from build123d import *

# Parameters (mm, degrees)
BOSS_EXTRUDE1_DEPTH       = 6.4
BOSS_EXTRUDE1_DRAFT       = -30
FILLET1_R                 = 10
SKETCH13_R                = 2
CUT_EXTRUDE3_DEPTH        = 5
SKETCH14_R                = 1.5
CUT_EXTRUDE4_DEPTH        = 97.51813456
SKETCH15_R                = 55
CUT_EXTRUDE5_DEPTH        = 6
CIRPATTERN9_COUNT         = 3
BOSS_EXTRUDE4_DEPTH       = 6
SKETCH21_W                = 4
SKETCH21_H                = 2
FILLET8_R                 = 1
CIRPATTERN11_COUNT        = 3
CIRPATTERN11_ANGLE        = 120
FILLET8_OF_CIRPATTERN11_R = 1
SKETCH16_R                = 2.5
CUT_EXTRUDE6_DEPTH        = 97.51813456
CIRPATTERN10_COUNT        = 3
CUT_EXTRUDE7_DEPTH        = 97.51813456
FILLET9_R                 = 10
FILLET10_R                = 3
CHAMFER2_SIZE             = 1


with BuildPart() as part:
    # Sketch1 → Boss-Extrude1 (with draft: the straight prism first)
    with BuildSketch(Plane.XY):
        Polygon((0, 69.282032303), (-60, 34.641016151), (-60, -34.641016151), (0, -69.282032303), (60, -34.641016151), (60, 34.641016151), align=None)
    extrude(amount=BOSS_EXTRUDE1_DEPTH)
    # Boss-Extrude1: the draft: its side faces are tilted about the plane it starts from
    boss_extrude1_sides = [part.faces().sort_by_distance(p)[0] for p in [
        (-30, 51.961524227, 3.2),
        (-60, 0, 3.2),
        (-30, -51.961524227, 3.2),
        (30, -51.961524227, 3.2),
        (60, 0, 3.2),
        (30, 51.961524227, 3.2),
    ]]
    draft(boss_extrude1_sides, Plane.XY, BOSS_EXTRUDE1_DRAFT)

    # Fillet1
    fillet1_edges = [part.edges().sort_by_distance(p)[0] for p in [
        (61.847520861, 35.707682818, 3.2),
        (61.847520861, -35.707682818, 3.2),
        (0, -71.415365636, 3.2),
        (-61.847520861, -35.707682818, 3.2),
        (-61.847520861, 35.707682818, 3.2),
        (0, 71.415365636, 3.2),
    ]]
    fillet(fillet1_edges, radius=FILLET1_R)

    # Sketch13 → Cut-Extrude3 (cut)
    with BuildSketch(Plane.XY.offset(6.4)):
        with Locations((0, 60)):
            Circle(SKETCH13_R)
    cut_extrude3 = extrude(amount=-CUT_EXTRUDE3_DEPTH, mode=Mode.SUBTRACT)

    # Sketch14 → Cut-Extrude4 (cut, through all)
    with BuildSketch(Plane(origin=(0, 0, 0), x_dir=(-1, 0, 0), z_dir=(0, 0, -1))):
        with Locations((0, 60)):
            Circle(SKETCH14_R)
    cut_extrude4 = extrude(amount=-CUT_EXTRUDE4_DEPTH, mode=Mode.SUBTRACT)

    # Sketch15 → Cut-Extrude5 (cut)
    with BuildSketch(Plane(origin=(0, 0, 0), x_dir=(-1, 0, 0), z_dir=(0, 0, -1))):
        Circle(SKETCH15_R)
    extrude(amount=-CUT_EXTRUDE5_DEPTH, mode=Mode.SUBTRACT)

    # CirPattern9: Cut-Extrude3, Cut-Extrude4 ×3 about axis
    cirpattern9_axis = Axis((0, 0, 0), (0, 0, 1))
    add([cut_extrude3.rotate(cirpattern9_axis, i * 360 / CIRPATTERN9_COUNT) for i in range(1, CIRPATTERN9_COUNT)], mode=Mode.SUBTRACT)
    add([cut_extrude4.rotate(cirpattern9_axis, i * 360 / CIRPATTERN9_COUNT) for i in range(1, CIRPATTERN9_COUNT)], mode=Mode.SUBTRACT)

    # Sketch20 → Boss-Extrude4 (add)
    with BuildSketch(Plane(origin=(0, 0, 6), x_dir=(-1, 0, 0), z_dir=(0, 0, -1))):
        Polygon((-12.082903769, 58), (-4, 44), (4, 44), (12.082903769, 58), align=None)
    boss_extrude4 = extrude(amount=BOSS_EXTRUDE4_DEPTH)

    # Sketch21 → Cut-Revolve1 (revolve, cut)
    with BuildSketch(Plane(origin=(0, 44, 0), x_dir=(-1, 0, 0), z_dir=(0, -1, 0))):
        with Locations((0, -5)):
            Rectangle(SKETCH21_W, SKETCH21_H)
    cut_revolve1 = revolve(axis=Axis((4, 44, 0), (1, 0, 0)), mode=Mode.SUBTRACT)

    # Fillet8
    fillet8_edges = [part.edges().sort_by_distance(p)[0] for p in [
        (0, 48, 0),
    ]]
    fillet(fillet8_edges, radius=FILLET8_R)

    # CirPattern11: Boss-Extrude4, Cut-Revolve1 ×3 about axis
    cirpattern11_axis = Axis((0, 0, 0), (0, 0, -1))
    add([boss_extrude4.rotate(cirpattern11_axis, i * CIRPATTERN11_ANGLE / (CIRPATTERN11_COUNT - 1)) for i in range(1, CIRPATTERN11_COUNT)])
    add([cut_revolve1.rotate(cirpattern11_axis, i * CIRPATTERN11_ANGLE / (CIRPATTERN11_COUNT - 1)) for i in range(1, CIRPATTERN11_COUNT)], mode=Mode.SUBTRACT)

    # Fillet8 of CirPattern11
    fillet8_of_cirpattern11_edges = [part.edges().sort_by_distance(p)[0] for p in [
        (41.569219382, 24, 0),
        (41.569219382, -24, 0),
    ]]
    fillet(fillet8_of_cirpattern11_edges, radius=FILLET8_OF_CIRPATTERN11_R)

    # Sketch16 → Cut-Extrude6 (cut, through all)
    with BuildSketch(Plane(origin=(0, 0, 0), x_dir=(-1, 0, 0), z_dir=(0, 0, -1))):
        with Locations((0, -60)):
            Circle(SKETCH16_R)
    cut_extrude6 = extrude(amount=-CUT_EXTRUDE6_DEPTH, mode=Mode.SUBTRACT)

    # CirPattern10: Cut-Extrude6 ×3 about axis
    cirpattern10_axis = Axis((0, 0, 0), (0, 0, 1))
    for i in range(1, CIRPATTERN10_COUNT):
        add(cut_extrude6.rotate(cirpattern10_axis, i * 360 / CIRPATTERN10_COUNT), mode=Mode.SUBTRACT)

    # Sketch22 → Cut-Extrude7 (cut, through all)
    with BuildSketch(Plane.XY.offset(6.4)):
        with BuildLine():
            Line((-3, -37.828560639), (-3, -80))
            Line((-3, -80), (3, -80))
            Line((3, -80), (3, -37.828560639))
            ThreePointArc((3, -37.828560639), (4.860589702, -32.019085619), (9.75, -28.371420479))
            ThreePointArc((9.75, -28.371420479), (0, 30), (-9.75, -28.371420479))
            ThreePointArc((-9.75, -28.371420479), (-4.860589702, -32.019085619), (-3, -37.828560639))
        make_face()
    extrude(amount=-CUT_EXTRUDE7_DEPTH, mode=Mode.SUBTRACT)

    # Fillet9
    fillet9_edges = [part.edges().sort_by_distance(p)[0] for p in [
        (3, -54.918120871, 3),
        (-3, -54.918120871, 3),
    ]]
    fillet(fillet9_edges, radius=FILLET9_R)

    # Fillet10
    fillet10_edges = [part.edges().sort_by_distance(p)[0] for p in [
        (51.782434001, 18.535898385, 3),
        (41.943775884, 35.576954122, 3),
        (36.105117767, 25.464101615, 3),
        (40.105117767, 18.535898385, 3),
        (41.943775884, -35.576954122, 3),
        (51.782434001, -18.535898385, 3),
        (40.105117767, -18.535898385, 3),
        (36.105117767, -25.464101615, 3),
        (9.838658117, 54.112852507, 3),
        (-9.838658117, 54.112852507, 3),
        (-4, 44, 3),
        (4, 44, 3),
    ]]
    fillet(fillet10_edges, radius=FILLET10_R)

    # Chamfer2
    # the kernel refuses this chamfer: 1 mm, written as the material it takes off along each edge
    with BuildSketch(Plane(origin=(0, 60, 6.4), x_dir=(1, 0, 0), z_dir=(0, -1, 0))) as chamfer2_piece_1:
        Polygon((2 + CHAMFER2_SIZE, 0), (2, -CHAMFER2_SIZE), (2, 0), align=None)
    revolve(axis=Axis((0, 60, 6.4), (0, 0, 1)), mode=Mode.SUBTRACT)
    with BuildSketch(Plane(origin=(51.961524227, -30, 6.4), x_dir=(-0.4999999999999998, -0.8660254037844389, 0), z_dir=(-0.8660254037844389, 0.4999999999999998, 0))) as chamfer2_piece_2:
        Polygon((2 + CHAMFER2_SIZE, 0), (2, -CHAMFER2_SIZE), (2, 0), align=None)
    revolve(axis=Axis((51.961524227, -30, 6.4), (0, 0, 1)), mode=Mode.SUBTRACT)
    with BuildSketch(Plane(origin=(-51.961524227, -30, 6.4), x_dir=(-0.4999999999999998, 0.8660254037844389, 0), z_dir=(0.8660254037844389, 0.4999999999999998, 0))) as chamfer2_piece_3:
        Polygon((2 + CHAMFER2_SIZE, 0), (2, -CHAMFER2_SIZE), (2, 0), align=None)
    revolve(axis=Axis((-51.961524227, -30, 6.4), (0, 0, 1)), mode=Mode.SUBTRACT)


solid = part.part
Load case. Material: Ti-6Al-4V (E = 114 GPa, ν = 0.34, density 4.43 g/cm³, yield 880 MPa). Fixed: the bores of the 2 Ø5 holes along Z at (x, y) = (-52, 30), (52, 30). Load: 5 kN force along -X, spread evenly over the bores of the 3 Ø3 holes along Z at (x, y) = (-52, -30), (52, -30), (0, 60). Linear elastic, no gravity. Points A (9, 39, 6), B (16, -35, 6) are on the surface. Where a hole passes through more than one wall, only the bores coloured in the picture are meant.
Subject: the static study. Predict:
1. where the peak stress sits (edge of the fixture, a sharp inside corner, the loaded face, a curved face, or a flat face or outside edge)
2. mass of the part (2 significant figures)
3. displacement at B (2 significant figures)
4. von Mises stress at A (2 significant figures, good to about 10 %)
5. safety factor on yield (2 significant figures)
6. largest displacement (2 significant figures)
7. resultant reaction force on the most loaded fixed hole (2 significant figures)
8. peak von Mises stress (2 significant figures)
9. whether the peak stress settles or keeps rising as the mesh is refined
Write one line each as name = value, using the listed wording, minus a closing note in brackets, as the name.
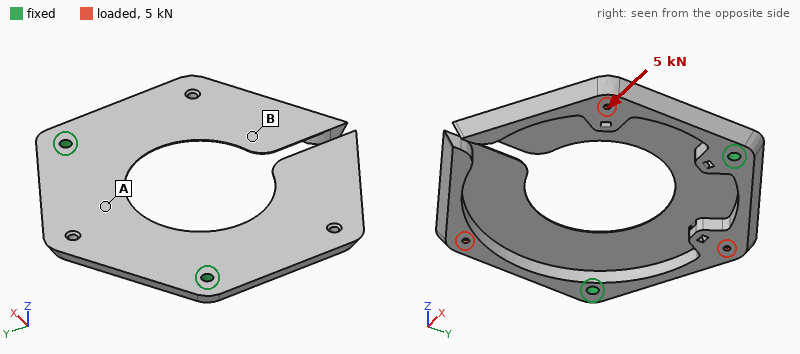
where the peak stress sits = a curved face
mass of the part = 120 g
displacement at B = 0.75 mm
von Mises stress at A = 160 MPa
safety factor on yield = 1.2
largest displacement = 1.2 mm
resultant reaction force on the most loaded fixed hole = 2.6 kN
peak von Mises stress = 710 MPa
whether the peak stress settles or keeps rising as the mesh is refined = settles
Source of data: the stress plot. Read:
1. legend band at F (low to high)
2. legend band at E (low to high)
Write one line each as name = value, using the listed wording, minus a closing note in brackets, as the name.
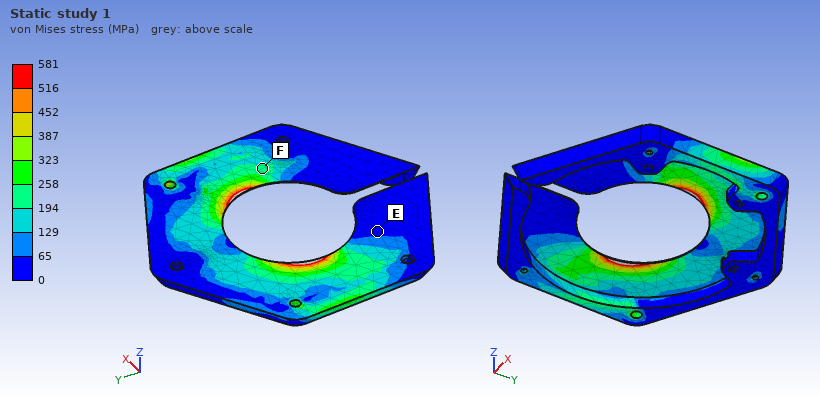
legend band at F = 194 to 258 MPa
legend band at E = 0 to 65 MPa
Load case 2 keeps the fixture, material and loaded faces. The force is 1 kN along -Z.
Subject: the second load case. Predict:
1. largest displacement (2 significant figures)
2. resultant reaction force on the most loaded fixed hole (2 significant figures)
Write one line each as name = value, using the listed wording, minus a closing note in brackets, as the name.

largest displacement = 2.3 mm
resultant reaction force on the most loaded fixed hole = 510 N
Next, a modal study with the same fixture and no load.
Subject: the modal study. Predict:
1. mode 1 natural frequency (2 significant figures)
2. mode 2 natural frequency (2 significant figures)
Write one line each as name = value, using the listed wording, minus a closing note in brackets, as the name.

mode 1 natural frequency = 370 Hz
mode 2 natural frequency = 370 Hz
